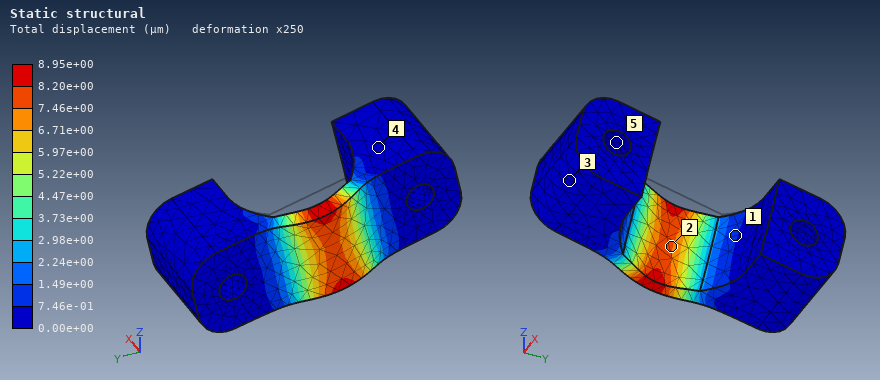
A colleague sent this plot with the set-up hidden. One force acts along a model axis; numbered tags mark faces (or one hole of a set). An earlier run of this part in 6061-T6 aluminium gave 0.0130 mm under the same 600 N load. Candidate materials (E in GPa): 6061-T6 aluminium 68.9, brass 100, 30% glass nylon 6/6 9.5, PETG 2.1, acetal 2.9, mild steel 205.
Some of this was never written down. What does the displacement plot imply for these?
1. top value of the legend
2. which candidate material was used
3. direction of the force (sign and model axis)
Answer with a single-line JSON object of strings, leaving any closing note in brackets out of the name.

{"top value of the legend": "8.95e+00 µm", "which candidate material was used": "brass", "direction of the force": "-X"}
